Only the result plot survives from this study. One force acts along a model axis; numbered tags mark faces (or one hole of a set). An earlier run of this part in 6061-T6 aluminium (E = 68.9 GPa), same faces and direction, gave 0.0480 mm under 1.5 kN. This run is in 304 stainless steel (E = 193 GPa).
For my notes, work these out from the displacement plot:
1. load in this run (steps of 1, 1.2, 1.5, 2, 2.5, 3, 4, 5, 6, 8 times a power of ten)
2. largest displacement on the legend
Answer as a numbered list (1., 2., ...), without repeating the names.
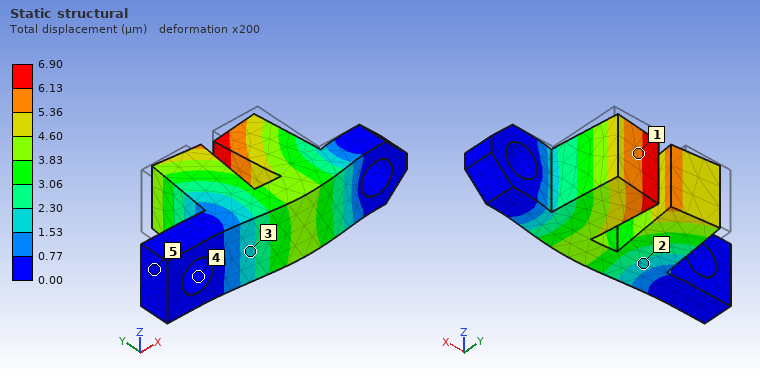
1. 600 N
2. 6.90 µm
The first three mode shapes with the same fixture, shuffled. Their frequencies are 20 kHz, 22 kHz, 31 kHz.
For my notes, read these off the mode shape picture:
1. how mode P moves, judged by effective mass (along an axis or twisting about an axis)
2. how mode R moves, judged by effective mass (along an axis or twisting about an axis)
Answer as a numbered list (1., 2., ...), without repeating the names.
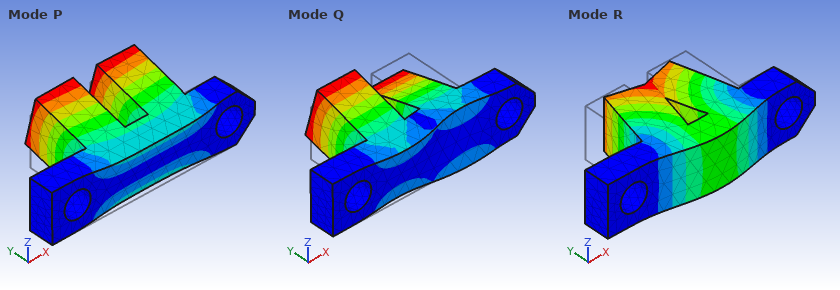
1. along Z
2. along Y
